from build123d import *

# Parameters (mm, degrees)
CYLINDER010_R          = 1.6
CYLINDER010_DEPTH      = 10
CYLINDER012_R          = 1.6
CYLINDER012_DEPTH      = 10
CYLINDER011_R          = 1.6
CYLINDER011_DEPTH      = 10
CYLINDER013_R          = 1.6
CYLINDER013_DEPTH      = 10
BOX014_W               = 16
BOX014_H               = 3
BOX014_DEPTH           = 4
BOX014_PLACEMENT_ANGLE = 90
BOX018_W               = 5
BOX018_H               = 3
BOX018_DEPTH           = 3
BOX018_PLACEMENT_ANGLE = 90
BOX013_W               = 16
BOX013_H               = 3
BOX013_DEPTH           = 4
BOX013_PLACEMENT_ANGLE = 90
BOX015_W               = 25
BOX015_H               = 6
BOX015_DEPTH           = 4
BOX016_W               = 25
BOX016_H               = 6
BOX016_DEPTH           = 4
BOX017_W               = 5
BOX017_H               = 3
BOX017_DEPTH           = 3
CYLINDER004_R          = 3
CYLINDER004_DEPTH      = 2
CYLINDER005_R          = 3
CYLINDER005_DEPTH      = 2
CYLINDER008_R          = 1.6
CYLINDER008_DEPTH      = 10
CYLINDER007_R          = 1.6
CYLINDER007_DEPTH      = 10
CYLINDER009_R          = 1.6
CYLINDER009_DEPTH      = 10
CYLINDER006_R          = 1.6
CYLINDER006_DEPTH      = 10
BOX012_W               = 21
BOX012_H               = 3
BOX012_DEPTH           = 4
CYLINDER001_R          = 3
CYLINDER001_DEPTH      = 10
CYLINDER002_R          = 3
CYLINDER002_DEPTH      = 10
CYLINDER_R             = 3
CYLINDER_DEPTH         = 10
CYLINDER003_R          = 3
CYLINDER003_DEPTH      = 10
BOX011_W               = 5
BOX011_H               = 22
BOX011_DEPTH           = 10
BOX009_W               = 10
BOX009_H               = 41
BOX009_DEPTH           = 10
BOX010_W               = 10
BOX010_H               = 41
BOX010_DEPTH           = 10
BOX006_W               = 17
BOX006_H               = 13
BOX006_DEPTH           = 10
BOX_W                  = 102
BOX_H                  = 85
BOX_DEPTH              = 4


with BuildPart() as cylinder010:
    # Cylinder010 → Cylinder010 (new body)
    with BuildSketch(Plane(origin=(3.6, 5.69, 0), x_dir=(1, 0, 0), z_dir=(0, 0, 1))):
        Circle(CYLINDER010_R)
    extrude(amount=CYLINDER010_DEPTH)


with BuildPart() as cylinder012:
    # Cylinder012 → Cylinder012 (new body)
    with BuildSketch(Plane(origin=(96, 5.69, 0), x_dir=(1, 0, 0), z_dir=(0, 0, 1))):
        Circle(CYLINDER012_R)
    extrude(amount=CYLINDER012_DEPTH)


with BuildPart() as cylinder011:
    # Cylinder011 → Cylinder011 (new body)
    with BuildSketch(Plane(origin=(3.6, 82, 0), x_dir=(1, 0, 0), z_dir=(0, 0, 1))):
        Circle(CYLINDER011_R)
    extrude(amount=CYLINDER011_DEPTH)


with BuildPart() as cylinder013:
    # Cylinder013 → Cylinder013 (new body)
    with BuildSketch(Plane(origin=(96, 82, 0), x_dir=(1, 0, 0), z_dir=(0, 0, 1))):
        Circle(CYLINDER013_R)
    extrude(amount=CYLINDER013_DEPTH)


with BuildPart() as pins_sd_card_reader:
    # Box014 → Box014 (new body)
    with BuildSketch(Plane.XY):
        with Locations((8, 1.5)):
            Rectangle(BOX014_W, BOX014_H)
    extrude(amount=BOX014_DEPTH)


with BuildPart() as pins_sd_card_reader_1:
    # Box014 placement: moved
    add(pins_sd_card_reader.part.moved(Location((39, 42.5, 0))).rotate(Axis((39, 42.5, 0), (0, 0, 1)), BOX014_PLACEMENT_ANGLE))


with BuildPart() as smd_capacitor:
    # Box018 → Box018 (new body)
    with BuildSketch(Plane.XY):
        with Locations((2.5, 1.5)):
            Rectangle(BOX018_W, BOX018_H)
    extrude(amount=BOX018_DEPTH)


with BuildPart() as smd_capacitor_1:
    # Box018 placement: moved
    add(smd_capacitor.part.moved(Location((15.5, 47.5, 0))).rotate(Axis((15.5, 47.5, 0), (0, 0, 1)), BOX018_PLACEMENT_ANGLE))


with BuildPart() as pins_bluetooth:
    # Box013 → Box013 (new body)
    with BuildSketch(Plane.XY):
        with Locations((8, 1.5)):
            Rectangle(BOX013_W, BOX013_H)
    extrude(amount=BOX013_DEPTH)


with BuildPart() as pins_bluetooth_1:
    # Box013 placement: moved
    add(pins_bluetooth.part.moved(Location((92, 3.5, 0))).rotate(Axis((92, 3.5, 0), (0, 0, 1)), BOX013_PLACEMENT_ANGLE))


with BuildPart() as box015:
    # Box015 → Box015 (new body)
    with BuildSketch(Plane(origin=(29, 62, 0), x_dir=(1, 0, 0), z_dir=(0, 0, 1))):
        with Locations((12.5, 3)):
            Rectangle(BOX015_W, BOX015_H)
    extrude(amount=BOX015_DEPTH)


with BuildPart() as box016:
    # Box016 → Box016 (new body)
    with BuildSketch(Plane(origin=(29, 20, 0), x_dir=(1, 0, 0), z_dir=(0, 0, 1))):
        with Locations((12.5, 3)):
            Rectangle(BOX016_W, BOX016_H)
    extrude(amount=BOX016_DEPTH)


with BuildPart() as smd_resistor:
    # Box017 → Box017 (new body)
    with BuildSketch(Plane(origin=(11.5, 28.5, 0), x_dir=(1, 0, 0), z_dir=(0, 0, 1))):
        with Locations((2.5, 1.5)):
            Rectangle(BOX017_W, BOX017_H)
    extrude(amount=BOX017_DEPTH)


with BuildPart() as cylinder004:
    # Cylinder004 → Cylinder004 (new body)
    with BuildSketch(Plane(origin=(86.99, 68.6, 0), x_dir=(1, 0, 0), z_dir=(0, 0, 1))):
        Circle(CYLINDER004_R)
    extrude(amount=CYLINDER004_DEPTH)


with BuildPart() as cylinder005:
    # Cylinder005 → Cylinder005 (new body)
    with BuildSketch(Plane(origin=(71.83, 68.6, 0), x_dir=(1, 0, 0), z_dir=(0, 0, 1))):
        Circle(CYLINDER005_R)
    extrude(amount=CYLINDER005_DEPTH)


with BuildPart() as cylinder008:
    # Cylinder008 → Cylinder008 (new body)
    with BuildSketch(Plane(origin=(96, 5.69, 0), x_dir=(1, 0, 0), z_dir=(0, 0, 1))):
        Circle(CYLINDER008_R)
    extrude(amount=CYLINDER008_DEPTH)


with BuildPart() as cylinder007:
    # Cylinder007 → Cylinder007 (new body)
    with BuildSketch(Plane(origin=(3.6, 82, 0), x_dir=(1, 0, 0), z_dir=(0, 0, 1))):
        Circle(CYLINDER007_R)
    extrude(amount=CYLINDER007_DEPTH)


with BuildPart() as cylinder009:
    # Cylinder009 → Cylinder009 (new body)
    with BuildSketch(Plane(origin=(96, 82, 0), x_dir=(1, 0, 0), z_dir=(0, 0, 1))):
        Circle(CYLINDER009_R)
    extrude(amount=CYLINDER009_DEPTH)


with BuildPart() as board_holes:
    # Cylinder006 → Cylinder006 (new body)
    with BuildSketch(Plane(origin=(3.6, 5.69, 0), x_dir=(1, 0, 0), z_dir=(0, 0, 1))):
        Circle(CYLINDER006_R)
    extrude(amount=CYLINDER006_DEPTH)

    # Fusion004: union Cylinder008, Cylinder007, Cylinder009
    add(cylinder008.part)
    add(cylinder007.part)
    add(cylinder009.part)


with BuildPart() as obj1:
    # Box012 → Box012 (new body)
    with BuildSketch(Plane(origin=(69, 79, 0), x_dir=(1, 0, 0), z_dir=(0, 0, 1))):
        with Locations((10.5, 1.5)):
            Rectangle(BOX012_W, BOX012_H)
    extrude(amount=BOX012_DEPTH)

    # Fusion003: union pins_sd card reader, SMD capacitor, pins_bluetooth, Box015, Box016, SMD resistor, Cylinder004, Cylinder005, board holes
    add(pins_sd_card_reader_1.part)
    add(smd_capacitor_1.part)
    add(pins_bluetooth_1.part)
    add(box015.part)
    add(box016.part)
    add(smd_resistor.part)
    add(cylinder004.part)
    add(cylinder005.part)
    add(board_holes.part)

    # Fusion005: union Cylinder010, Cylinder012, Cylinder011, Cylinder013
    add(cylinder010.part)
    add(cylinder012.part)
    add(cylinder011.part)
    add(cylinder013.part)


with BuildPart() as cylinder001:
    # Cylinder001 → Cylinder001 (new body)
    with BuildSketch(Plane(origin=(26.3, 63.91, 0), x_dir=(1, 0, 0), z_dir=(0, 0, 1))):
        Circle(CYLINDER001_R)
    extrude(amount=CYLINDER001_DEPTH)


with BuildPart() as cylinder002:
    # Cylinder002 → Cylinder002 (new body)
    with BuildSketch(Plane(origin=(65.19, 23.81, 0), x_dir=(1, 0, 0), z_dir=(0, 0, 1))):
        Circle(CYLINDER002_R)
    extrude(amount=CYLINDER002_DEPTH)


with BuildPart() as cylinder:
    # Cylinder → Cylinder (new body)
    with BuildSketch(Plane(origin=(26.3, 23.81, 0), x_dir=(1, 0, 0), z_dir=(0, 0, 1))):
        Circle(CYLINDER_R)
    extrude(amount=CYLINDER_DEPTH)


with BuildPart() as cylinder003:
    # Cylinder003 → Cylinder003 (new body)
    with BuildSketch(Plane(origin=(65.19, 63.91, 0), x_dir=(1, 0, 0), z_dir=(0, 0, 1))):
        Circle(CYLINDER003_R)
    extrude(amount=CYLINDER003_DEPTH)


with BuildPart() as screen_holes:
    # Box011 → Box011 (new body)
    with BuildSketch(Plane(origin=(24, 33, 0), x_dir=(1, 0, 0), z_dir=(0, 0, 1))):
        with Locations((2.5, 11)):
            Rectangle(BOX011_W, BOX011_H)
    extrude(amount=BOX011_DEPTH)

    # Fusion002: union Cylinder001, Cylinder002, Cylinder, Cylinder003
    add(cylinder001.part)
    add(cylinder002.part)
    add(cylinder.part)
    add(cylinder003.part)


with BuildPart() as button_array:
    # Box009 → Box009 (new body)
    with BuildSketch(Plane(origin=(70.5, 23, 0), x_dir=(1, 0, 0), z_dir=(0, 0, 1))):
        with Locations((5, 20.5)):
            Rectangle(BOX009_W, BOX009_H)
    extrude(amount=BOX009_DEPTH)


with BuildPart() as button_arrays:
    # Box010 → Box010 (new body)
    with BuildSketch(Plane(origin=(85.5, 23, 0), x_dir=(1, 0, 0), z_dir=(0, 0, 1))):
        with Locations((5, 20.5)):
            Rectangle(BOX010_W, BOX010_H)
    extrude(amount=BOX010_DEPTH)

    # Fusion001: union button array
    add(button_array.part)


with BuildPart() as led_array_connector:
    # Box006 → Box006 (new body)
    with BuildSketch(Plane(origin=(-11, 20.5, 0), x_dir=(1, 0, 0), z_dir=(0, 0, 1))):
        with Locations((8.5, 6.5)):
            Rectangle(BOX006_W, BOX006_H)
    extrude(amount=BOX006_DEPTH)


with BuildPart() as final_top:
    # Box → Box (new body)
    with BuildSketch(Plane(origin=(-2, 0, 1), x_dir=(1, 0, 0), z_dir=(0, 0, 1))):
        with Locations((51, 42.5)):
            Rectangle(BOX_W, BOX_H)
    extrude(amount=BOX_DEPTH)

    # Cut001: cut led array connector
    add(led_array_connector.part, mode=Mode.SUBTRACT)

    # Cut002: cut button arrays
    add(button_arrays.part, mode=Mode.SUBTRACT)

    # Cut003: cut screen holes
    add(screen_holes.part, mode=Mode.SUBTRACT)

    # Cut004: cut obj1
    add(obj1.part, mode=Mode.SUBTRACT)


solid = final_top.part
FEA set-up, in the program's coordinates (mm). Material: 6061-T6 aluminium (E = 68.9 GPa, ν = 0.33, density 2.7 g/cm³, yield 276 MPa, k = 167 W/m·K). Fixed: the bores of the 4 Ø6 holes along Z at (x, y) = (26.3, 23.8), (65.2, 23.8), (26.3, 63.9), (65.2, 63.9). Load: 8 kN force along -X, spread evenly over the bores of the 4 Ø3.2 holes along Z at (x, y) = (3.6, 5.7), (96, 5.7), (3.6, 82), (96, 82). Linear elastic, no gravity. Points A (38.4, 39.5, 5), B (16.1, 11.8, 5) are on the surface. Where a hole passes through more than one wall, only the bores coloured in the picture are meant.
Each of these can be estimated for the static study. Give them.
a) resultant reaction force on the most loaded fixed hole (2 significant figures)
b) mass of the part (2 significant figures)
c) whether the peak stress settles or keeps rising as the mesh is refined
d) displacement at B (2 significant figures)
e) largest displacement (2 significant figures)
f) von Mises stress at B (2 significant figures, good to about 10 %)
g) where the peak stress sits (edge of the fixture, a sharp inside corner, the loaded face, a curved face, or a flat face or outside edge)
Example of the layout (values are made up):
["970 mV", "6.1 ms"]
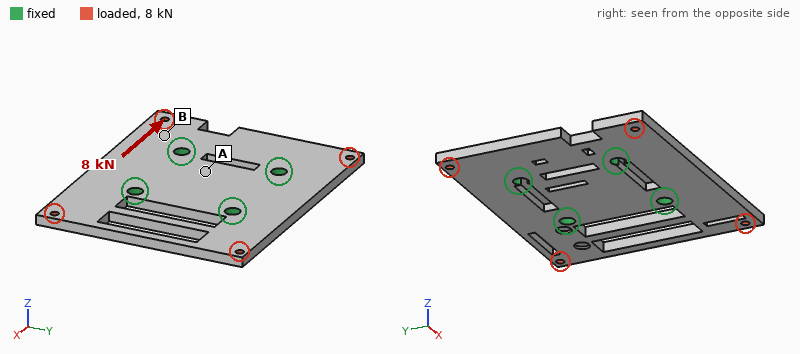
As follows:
["2.3 kN", "77 g", "keeps rising", "12 µm", "61 µm", "29 MPa", "a sharp inside corner"]
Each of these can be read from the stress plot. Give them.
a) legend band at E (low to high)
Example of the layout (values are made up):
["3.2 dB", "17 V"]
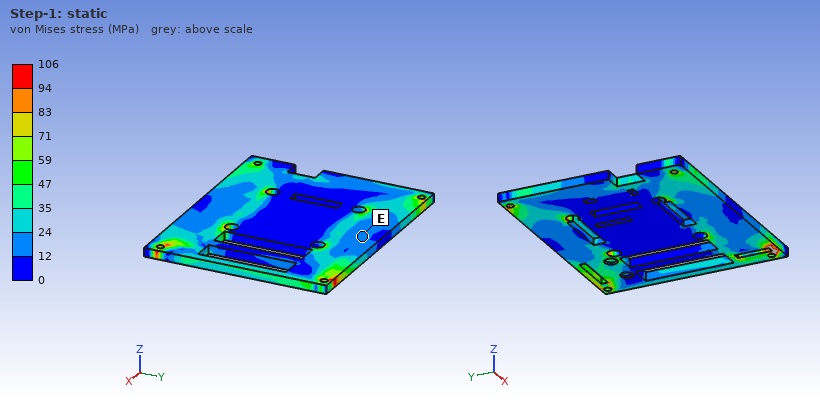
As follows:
["12 to 24 MPa"]
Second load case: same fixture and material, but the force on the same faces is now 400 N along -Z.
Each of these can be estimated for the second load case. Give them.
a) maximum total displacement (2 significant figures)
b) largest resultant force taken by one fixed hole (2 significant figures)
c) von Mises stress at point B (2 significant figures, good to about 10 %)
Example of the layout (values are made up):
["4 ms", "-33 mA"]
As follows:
["0.24 mm", "110 N", "16 MPa"]
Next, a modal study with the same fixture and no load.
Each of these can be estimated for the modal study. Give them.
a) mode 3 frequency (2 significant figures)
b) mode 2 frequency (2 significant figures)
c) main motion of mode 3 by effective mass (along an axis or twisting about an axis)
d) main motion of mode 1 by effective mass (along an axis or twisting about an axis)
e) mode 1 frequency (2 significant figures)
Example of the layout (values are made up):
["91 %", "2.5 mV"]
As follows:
["3800 Hz", "2600 Hz", "along Z", "along Z", "2000 Hz"]
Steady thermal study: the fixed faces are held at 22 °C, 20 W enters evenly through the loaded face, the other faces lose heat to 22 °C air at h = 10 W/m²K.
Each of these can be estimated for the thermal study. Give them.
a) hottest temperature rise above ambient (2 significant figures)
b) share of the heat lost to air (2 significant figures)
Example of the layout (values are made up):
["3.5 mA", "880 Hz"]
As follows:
["18 K", "3.8 %"]
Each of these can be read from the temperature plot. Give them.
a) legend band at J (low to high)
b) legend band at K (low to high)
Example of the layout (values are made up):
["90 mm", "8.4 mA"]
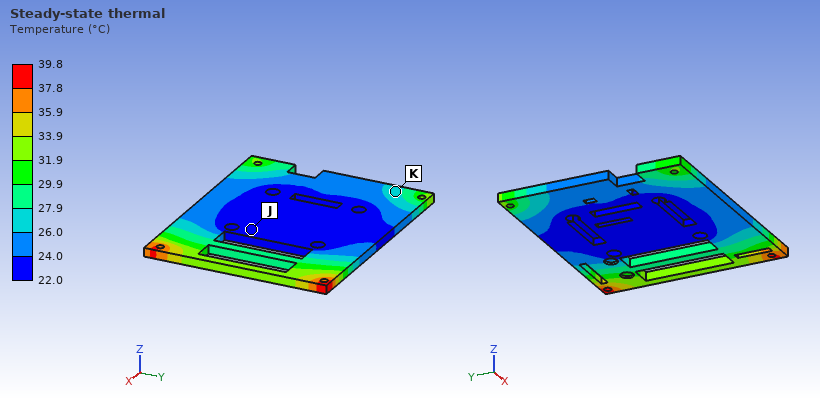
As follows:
["22.0 to 24.0 °C", "26.0 to 27.9 °C"]
